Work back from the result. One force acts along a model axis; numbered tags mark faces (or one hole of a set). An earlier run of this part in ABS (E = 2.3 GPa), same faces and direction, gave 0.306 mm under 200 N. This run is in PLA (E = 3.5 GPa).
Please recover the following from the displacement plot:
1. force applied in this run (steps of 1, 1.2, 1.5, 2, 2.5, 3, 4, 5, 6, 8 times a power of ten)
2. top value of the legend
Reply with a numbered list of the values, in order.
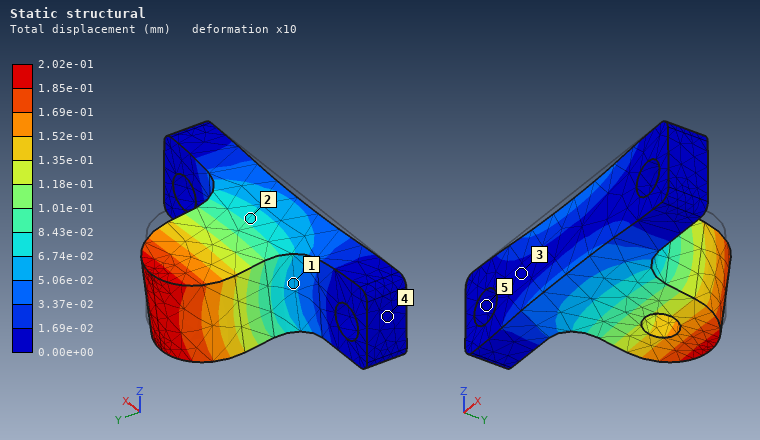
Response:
1. 200 N
2. 2.02e-01 mm
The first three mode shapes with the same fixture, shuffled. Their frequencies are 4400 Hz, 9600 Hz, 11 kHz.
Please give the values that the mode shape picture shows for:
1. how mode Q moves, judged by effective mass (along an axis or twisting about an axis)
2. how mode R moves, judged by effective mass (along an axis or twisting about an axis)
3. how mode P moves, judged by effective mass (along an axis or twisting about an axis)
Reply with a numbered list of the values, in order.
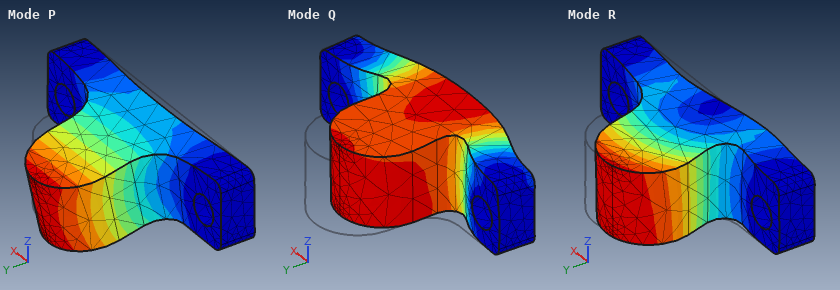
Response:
1. along Y
2. along X
3. along Z
